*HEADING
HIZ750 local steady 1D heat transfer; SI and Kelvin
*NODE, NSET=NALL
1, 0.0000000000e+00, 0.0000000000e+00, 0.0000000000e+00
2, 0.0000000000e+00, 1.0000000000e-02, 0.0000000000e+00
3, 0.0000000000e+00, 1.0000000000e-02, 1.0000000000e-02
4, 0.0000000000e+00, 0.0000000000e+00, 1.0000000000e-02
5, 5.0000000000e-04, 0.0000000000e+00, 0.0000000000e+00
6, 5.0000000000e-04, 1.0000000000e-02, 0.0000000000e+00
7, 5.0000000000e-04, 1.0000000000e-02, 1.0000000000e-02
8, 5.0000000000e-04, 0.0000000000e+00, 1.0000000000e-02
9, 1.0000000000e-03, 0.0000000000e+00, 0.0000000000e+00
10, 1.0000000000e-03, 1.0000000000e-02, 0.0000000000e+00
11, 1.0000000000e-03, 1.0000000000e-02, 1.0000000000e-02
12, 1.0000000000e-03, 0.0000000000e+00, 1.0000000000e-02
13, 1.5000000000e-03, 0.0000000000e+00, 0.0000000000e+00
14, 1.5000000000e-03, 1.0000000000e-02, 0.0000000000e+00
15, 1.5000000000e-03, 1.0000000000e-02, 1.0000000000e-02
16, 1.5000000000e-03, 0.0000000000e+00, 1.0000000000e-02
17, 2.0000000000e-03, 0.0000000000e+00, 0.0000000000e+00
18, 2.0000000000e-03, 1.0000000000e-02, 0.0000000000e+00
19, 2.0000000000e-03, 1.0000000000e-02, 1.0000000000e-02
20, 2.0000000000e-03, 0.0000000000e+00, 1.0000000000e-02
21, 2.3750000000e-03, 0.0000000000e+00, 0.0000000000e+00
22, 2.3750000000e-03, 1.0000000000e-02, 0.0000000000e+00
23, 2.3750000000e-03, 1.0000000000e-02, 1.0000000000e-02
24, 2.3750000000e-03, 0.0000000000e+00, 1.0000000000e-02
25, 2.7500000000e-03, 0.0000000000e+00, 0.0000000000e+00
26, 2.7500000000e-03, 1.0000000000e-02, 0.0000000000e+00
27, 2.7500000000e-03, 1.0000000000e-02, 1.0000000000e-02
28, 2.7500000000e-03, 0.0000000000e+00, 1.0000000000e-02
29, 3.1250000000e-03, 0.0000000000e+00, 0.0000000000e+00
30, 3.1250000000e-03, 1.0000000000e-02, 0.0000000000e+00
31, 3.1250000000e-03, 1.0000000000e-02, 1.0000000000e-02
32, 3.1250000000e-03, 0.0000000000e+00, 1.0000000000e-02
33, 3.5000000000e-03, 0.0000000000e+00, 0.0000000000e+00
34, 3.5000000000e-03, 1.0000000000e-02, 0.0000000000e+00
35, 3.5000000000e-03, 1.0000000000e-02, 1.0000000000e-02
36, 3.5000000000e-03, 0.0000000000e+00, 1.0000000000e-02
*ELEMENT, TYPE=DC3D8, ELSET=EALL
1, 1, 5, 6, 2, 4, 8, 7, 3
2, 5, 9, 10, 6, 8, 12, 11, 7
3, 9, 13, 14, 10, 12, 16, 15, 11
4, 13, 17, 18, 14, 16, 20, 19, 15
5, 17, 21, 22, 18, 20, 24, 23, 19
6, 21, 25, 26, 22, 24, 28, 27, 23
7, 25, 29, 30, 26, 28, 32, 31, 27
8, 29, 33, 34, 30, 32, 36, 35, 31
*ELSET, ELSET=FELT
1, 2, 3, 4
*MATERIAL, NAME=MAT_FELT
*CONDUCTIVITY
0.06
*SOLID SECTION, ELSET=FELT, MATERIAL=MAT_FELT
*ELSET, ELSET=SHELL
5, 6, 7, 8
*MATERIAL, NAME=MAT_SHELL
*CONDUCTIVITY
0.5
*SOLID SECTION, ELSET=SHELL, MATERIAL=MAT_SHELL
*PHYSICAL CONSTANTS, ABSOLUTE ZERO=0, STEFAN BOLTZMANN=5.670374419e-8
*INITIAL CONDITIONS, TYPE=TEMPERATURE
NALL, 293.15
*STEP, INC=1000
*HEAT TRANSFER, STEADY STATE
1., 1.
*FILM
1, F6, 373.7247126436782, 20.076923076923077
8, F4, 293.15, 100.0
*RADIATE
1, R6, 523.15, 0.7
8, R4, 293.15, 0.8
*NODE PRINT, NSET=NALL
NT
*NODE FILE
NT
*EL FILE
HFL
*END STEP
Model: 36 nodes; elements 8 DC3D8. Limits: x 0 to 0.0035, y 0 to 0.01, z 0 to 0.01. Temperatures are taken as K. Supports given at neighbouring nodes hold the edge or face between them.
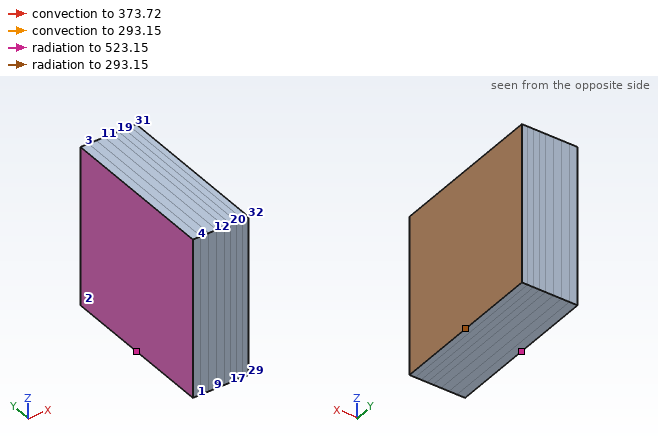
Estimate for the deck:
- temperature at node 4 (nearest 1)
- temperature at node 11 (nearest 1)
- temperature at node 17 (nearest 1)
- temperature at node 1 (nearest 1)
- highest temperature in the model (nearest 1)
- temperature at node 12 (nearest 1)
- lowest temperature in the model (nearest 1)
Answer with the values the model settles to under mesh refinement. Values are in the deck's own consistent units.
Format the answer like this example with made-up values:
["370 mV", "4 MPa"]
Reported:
["382 K", "350 K", "318 K", "382 K", "382 K", "350 K", "312 K"]
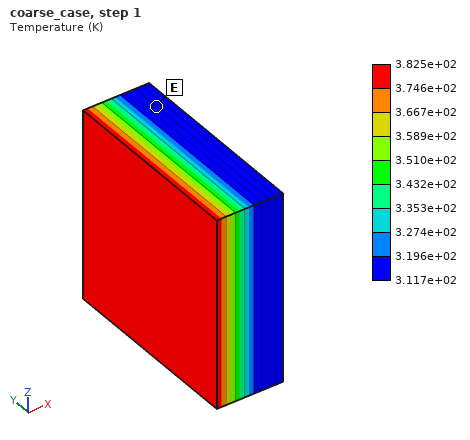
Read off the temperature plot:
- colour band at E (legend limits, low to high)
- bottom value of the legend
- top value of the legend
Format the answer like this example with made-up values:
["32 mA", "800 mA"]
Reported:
["3.117e+02 to 3.196e+02 K", "3.117e+02 K", "3.825e+02 K"]
